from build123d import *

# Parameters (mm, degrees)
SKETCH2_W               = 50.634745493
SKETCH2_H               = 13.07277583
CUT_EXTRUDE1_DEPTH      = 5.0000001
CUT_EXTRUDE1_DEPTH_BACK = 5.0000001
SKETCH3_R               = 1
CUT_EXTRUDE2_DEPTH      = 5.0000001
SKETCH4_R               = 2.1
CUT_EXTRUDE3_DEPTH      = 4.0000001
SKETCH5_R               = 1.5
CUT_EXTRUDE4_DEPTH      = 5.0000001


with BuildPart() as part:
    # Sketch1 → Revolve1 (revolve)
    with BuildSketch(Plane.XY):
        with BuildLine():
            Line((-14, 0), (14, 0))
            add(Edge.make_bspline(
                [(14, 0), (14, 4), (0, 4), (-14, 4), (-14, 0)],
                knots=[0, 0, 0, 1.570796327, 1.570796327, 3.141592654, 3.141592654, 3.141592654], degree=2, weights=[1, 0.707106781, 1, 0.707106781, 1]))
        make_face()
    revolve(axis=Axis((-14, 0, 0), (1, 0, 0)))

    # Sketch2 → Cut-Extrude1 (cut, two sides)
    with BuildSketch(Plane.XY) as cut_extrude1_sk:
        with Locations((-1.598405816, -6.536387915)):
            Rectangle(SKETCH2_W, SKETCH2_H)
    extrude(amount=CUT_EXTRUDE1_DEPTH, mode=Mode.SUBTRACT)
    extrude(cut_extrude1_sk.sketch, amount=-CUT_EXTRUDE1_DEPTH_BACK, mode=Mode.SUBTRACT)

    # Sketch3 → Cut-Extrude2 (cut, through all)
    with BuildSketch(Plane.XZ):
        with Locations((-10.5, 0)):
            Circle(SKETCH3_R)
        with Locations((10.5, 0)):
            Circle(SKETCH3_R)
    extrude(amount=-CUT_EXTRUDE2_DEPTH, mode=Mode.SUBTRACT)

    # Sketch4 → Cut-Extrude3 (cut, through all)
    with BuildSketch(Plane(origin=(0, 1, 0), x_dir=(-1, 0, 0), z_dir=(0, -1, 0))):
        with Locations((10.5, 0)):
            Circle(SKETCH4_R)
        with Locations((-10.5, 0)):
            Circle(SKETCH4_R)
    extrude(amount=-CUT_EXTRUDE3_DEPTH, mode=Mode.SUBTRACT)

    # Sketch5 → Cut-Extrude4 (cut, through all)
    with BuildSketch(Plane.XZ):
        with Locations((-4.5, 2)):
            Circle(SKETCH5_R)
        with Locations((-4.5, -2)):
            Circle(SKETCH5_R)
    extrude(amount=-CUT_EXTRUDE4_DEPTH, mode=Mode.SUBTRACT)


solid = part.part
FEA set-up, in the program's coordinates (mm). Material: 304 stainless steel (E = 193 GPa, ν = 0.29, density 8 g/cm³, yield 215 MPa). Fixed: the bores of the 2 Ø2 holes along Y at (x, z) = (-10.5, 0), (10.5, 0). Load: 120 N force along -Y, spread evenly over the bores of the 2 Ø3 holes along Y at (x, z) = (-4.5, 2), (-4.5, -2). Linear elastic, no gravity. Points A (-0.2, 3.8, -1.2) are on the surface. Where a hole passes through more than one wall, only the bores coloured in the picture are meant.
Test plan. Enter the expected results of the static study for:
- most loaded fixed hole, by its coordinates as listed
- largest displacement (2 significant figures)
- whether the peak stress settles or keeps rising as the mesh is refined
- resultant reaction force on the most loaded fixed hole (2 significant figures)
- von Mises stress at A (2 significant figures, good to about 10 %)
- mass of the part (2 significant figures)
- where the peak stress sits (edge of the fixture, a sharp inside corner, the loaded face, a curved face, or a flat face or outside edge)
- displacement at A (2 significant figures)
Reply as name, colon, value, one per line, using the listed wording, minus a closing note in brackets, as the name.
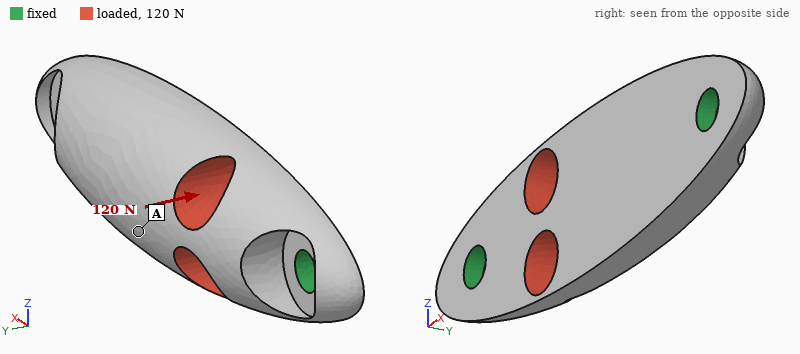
most loaded fixed hole, by its coordinates as listed: (-10.5, 0)
largest displacement: 4.0 µm
whether the peak stress settles or keeps rising as the mesh is refined: keeps rising
resultant reaction force on the most loaded fixed hole: 130 N
von Mises stress at A: 18 MPa
mass of the part: 3.1 g
where the peak stress sits: edge of the fixture
displacement at A: 3.1 µm
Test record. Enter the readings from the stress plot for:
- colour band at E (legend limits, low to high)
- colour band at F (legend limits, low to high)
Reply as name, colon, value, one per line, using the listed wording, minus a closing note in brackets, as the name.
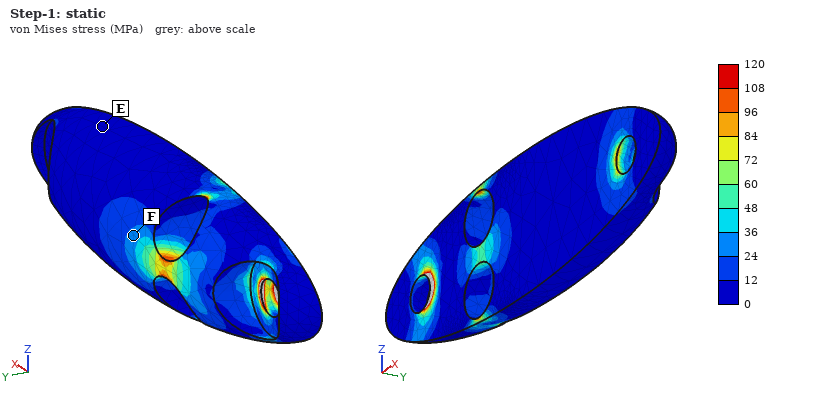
colour band at E: 0 to 12 MPa
colour band at F: 24 to 36 MPa
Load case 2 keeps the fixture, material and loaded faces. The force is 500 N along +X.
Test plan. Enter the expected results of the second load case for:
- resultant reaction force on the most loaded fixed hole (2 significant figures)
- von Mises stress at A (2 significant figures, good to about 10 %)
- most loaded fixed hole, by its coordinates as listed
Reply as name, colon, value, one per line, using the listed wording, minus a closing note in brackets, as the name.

resultant reaction force on the most loaded fixed hole: 270 N
von Mises stress at A: 8.0 MPa
most loaded fixed hole, by its coordinates as listed: (-10.5, 0)
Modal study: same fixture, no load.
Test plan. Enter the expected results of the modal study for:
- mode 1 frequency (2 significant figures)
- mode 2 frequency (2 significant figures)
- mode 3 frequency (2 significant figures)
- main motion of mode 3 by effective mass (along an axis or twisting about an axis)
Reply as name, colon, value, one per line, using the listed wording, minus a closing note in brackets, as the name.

mode 1 frequency: 21 kHz
mode 2 frequency: 22 kHz
mode 3 frequency: 29 kHz
main motion of mode 3 by effective mass: along Z
